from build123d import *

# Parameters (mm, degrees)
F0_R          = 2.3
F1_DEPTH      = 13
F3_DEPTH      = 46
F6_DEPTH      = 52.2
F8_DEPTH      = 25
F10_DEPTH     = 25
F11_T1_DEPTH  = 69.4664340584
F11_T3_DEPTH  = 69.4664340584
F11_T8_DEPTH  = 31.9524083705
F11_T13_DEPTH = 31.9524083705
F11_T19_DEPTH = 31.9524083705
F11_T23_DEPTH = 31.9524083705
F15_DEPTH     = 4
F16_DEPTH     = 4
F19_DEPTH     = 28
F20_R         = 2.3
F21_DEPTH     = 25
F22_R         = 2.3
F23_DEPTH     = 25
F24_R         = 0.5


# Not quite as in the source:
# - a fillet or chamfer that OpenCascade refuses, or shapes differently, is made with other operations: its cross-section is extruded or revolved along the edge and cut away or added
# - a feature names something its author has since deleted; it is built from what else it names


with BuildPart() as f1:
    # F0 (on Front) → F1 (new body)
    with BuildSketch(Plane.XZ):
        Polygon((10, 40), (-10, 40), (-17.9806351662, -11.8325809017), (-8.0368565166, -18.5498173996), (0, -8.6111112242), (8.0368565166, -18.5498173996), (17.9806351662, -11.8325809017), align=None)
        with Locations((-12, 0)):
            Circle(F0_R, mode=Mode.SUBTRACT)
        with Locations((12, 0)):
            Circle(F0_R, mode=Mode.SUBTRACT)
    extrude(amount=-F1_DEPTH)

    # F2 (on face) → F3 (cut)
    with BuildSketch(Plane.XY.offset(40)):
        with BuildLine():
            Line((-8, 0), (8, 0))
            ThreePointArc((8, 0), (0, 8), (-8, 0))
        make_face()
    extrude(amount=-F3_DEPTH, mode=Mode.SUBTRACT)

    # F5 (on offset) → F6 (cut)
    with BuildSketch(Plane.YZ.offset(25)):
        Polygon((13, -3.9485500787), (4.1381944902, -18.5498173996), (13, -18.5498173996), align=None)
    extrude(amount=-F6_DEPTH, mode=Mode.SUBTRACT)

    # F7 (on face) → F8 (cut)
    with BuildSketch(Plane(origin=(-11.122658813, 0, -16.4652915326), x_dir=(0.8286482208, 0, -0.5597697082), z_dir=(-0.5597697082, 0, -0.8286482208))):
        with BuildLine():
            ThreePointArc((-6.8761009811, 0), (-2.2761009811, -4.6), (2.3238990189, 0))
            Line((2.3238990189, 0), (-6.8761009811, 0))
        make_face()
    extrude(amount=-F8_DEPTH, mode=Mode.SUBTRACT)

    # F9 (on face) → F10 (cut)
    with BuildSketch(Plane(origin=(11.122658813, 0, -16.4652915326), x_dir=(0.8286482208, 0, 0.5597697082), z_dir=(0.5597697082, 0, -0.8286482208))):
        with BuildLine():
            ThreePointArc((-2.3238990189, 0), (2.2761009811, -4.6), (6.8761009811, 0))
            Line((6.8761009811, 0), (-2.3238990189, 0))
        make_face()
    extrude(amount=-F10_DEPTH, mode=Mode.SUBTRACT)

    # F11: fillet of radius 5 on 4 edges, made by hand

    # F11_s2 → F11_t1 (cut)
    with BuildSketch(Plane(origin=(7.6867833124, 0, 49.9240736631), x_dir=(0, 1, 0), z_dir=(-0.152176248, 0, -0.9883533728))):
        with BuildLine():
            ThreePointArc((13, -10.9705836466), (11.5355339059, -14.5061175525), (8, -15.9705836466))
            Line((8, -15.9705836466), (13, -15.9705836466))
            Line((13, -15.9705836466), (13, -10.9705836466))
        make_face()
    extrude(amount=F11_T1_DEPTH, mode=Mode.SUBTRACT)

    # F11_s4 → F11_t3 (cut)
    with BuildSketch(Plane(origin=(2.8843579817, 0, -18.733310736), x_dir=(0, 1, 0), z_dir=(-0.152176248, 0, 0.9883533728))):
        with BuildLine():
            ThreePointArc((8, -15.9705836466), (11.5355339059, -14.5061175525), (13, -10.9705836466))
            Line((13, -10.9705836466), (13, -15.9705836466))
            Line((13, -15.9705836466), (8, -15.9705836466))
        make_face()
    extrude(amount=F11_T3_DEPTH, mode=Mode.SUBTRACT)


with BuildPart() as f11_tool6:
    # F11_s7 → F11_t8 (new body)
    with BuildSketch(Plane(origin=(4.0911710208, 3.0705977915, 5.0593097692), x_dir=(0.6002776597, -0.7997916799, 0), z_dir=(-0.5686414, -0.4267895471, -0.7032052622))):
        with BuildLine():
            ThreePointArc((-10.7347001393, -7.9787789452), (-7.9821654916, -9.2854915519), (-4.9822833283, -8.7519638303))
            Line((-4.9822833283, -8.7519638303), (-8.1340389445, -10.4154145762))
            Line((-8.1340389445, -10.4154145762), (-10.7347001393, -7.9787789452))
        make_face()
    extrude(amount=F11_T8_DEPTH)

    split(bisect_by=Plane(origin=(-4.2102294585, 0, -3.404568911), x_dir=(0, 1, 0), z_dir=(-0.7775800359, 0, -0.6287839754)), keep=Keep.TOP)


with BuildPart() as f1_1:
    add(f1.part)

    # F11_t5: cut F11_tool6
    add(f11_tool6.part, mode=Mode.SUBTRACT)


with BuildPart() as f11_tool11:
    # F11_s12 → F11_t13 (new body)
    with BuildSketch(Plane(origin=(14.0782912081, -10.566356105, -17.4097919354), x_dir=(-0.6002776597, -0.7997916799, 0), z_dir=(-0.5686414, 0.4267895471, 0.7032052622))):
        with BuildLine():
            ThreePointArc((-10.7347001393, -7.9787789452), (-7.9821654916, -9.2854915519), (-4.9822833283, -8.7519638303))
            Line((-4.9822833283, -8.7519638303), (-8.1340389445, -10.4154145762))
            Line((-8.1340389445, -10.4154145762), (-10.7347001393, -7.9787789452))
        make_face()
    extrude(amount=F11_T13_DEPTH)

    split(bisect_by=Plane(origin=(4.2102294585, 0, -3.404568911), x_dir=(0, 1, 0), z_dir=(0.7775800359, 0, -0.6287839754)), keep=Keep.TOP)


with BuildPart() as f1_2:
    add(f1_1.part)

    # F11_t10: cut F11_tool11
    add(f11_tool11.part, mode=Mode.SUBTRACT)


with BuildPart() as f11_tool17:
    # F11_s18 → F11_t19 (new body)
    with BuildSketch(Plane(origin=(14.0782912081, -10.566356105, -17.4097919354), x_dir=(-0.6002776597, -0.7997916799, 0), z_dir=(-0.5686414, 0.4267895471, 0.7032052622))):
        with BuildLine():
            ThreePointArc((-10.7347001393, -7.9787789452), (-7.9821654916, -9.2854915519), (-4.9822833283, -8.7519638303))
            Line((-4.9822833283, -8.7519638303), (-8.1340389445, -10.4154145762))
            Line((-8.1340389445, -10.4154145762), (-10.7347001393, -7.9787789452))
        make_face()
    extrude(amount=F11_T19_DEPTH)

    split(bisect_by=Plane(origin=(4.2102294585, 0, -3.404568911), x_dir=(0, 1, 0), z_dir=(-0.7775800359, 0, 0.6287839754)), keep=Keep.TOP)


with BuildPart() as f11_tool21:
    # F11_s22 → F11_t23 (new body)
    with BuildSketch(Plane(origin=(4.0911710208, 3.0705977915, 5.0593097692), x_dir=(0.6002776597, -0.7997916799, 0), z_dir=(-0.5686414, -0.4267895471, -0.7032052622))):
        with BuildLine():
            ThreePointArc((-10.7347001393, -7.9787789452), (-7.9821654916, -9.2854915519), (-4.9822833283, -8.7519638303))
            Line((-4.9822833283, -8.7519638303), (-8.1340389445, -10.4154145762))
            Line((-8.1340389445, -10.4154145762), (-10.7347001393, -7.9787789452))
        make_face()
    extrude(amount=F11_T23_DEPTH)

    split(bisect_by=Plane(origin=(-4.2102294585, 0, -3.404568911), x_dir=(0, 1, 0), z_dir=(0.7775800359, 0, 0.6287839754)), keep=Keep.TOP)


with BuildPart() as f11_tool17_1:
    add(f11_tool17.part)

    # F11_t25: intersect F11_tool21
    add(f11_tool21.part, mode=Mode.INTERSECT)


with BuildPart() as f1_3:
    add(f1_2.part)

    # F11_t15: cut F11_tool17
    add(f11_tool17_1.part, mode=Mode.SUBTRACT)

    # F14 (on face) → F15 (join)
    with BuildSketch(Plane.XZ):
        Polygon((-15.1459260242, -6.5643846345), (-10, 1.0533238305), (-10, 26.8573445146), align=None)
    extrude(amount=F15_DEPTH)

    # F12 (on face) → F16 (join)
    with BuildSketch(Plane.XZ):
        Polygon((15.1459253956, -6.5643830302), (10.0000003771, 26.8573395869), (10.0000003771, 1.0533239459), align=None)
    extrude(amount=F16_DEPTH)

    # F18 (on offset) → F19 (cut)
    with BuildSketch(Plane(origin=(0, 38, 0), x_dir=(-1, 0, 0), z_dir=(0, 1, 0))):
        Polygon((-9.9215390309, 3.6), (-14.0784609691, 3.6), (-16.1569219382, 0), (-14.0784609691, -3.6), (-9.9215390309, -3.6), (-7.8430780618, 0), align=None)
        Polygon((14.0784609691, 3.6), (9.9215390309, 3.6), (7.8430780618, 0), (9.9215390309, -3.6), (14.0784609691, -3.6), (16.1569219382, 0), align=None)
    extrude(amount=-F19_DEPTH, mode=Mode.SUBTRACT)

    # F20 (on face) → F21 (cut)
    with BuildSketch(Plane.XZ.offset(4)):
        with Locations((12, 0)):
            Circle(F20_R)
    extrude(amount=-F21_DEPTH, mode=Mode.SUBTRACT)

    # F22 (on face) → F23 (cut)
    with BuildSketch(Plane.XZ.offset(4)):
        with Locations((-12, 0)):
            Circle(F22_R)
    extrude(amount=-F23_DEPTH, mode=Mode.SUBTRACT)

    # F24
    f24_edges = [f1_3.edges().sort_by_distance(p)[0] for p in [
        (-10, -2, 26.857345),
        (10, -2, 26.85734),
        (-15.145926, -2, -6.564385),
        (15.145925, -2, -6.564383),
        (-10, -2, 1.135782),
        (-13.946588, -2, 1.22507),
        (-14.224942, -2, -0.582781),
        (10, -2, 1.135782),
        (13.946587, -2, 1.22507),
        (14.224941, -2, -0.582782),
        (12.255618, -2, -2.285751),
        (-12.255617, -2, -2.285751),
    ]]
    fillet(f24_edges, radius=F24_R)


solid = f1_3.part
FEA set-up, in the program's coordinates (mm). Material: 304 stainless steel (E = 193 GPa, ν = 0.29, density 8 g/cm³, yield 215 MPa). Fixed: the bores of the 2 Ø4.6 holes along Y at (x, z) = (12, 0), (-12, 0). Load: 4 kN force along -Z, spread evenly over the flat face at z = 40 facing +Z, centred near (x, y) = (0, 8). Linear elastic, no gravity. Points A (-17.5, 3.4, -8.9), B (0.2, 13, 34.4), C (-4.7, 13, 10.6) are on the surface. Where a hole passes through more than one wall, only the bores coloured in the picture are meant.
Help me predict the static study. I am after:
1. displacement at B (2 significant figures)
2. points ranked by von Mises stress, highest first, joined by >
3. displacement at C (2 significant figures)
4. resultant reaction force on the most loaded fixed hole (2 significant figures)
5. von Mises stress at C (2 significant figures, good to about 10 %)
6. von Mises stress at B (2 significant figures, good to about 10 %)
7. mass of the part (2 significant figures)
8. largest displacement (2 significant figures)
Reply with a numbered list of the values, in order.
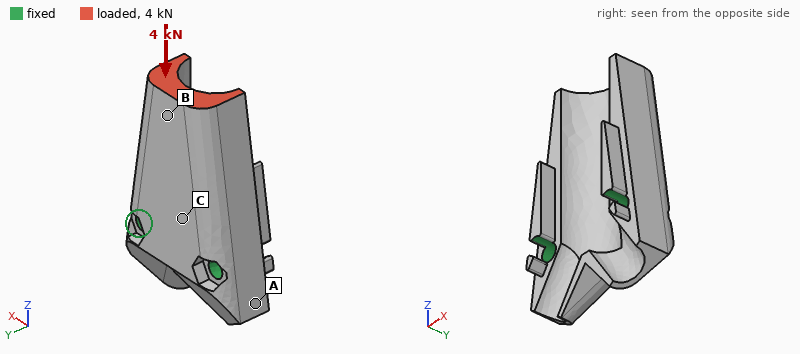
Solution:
1. 8.4 µm
2. B > C > A
3. 2.7 µm
4. 2.0 kN
5. 18 MPa
6. 28 MPa
7. 100 g
8. 10 µm
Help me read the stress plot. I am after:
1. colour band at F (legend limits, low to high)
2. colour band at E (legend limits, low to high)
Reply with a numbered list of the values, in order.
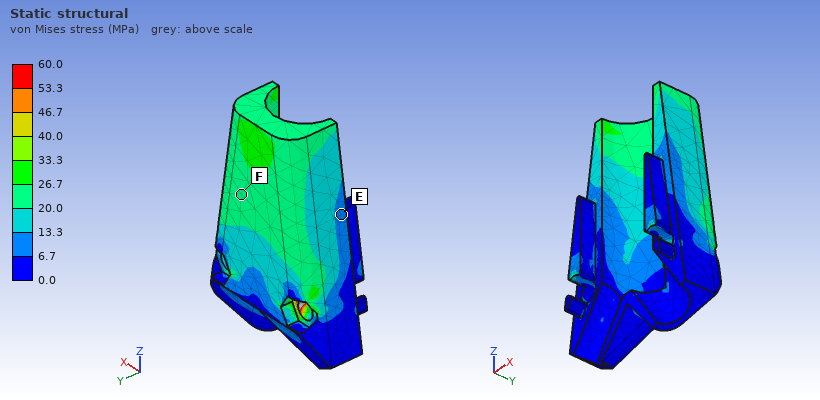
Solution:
1. 20.0 to 26.7 MPa
2. 6.7 to 13.3 MPa
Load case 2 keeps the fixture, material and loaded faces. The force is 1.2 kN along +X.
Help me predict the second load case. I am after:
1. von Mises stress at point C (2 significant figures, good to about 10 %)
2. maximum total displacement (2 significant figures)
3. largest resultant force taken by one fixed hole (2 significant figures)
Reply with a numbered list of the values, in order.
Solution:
1. 8.3 MPa
2. 21 µm
3. 1.9 kN
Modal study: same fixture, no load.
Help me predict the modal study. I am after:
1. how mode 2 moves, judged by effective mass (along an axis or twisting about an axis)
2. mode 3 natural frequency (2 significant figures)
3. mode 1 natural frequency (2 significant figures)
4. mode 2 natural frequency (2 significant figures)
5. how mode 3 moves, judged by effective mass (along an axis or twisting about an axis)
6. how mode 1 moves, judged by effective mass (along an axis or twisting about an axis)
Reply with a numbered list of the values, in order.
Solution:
1. along X
2. 18 kHz
3. 7300 Hz
4. 11 kHz
5. along X
6. along Y
